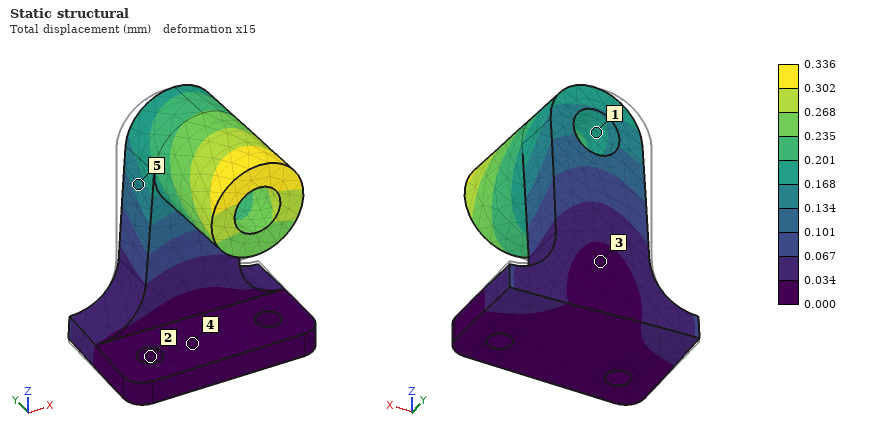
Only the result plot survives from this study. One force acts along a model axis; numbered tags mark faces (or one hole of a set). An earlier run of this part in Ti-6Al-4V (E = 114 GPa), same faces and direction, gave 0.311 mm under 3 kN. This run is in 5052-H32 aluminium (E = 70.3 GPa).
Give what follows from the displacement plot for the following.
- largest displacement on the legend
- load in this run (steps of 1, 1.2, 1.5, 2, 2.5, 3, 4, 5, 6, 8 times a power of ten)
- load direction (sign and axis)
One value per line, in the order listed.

0.336 mm
2 kN
+X
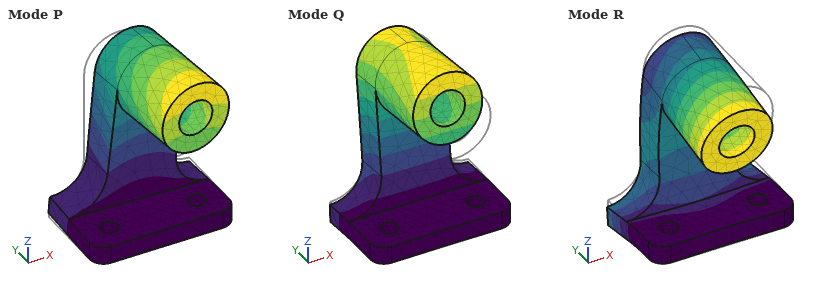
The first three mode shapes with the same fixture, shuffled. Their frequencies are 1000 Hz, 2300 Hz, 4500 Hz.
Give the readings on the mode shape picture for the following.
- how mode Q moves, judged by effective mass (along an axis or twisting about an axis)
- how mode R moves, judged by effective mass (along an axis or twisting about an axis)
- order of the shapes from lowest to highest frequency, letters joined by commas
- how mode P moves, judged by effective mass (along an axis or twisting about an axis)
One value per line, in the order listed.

along Y
along Z
Q, P, R
along X
